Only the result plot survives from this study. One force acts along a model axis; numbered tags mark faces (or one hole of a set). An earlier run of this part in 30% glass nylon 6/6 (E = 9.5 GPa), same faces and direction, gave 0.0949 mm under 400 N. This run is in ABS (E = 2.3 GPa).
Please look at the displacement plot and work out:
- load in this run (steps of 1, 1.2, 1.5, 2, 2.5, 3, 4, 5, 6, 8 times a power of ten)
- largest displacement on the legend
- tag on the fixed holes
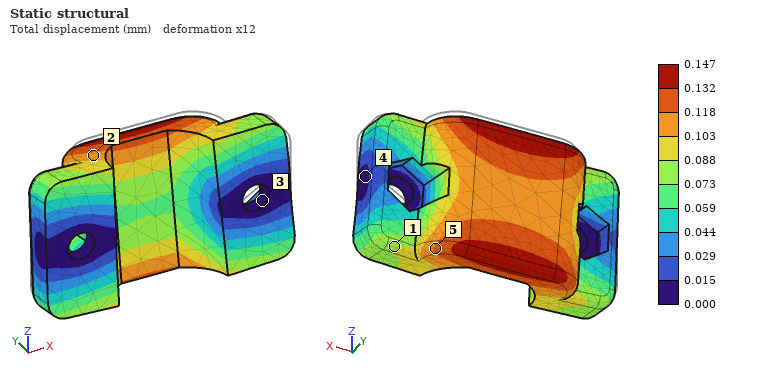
150 N
0.147 mm
3
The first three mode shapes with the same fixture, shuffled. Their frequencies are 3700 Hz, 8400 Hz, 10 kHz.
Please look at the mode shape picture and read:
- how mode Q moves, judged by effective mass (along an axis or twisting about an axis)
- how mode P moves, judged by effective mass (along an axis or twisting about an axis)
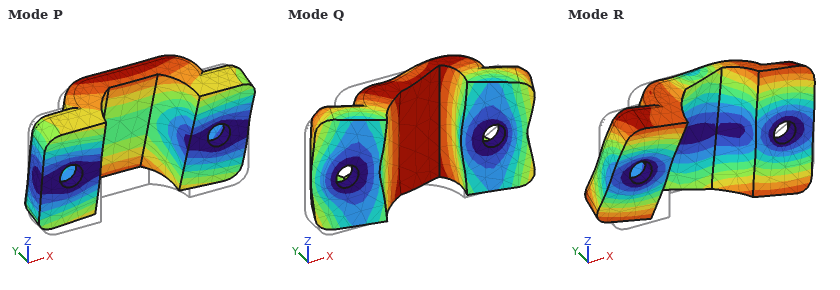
along X
along Z
